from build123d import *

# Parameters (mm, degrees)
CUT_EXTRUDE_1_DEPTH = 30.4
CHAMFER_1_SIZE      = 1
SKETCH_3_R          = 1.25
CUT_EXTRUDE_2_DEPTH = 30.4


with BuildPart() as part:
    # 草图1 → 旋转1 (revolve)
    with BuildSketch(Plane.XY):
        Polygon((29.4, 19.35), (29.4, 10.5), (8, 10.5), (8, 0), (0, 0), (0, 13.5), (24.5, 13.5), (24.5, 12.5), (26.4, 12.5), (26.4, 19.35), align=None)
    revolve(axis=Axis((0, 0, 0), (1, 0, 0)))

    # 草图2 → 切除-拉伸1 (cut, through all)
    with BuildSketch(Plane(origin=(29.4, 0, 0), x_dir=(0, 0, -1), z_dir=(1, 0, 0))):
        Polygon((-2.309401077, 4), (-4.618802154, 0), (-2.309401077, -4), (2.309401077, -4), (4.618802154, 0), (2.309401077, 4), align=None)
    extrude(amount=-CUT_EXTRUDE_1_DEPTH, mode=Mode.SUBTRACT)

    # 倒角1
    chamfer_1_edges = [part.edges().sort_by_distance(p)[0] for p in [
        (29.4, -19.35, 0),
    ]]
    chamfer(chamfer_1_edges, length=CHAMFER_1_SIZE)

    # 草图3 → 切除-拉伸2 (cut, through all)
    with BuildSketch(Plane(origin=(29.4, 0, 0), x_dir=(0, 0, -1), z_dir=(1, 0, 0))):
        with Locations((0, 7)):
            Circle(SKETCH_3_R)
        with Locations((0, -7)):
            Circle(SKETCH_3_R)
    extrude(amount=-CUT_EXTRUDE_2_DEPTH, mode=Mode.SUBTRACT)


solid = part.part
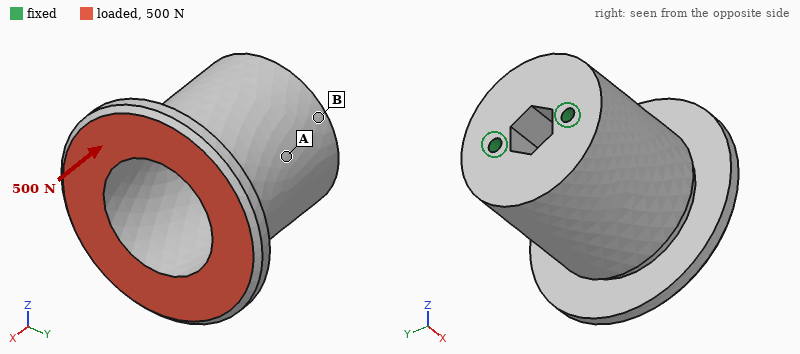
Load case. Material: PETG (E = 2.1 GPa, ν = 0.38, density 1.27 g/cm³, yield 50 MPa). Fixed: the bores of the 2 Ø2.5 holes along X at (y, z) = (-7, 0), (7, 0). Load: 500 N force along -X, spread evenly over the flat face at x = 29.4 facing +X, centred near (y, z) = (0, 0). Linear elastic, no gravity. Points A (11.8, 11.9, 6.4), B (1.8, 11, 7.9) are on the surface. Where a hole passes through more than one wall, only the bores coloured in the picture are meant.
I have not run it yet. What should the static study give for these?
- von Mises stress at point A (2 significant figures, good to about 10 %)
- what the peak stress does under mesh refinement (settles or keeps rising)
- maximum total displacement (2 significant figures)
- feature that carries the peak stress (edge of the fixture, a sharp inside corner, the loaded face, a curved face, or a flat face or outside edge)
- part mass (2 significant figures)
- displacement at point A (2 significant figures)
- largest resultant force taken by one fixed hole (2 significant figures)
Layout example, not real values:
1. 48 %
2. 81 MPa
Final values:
1. 2.6 MPa
2. keeps rising
3. 0.18 mm
4. edge of the fixture
5. 13 g
6. 0.030 mm
7. 250 N
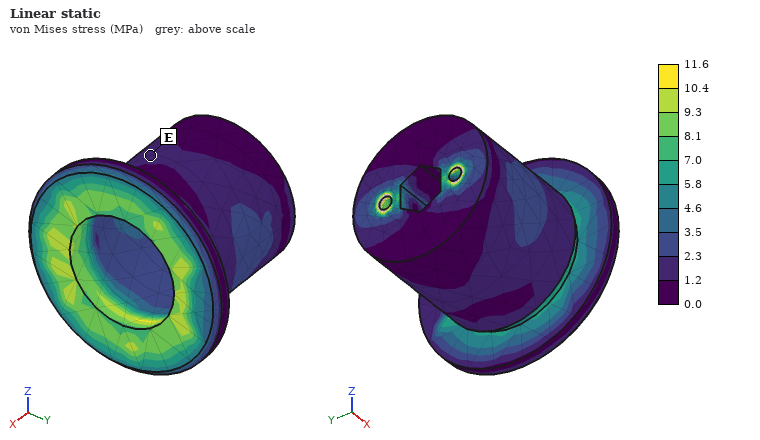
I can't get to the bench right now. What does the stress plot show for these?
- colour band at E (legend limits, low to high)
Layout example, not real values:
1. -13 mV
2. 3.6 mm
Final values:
1. 1.2 to 2.3 MPa
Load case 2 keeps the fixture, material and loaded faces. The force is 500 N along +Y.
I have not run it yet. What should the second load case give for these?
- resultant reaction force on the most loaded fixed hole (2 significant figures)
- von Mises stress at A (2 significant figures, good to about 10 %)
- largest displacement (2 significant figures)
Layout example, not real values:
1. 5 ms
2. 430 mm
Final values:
1. 660 N
2. 6.4 MPa
3. 0.50 mm
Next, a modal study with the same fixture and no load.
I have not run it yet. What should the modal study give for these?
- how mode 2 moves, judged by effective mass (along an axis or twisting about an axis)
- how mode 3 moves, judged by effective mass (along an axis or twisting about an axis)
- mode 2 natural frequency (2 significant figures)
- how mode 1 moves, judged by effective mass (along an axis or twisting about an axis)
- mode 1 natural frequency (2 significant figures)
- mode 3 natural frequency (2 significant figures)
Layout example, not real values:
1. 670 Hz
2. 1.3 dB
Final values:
1. along Y
2. twisting about X
3. 2600 Hz
4. along Z
5. 1800 Hz
6. 3900 Hz
